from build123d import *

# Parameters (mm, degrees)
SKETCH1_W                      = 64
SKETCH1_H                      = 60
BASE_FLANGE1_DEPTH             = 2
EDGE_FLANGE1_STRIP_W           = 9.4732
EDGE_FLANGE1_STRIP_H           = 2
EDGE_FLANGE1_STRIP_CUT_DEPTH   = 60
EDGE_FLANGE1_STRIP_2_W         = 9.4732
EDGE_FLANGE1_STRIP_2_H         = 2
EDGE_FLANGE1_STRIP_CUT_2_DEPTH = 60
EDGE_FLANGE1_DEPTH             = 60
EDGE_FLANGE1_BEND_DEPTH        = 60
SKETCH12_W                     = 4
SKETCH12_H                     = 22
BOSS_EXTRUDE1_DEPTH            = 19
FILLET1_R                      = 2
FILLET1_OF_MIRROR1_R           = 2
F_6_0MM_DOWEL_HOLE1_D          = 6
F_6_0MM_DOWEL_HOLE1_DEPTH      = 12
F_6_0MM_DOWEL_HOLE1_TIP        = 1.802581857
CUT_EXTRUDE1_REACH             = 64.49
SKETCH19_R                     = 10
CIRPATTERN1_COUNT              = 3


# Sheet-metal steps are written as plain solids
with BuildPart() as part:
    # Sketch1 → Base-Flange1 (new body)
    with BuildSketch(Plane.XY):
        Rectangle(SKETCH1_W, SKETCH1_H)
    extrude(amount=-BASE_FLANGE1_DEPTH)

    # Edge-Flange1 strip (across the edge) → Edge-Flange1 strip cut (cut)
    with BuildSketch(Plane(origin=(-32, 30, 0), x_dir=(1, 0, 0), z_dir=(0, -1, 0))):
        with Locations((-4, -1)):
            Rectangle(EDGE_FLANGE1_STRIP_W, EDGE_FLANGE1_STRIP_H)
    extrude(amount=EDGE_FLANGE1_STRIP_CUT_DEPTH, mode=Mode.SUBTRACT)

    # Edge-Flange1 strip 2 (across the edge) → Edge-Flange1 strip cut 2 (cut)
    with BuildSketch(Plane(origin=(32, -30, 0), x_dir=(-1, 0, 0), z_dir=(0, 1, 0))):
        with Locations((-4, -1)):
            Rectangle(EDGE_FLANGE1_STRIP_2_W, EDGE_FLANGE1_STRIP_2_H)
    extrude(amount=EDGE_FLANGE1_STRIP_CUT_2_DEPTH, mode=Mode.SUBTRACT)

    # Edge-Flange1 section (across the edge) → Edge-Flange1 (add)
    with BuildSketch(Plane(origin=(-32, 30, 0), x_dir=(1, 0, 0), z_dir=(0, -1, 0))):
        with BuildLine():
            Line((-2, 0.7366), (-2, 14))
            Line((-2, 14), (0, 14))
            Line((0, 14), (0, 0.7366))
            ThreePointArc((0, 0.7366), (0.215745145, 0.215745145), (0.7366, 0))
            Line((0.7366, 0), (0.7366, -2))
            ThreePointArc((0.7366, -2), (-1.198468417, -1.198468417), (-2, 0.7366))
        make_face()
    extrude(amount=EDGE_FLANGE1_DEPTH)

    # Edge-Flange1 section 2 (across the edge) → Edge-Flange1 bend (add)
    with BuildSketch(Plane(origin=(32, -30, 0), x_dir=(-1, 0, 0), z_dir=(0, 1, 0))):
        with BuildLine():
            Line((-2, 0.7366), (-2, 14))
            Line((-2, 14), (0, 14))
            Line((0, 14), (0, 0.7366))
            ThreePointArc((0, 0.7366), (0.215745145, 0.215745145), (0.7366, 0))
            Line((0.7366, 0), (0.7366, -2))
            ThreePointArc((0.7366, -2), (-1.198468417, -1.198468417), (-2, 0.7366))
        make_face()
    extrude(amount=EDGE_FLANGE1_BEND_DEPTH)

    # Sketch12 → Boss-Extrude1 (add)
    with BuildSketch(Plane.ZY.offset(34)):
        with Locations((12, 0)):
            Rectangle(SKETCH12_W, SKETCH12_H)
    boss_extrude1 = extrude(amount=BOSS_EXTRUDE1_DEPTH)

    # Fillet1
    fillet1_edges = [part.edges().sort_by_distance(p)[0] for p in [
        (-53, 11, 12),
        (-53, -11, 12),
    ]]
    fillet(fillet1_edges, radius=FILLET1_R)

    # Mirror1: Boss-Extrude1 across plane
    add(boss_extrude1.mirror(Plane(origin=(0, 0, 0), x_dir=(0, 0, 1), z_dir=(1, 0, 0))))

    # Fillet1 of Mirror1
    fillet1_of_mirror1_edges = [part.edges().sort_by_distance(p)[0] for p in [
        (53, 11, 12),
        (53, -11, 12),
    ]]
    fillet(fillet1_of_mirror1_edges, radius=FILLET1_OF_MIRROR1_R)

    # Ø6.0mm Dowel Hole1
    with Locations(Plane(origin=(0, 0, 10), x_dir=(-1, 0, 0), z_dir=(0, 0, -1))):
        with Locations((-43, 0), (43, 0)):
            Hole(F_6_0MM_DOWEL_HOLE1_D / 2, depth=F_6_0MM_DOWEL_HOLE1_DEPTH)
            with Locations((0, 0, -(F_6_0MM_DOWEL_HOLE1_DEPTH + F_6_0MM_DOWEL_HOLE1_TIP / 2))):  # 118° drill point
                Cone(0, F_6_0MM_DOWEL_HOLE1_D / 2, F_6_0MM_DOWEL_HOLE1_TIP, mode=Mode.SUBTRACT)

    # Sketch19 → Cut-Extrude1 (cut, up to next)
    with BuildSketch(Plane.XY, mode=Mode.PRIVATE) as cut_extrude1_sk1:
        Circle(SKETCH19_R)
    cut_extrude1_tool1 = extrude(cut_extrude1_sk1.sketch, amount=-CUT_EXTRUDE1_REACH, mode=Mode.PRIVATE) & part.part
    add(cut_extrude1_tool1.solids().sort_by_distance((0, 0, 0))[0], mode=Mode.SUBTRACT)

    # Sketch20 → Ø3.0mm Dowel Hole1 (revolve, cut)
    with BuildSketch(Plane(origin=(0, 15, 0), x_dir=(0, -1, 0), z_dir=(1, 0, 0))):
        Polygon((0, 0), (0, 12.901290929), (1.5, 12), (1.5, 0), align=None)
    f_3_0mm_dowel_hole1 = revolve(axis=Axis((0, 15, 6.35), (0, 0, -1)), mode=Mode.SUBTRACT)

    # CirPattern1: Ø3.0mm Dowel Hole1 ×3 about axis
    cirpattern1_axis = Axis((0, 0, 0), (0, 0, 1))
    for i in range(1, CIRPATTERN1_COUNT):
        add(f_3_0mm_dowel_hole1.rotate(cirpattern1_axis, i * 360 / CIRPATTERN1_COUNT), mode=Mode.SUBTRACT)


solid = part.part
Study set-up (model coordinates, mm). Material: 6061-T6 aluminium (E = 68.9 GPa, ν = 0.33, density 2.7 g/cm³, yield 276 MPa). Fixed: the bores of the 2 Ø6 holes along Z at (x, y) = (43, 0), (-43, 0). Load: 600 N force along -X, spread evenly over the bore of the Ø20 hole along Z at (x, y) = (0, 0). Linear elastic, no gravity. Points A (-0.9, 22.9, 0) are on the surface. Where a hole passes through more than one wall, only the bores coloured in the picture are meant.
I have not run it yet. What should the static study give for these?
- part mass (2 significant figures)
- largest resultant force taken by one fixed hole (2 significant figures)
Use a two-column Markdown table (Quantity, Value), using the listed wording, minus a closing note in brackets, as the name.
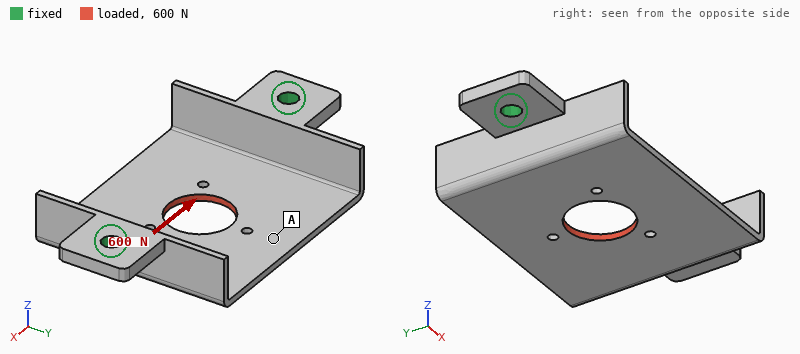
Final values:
| Quantity | Value |
|---|---|
| part mass | 37 g |
| largest resultant force taken by one fixed hole | 300 N |
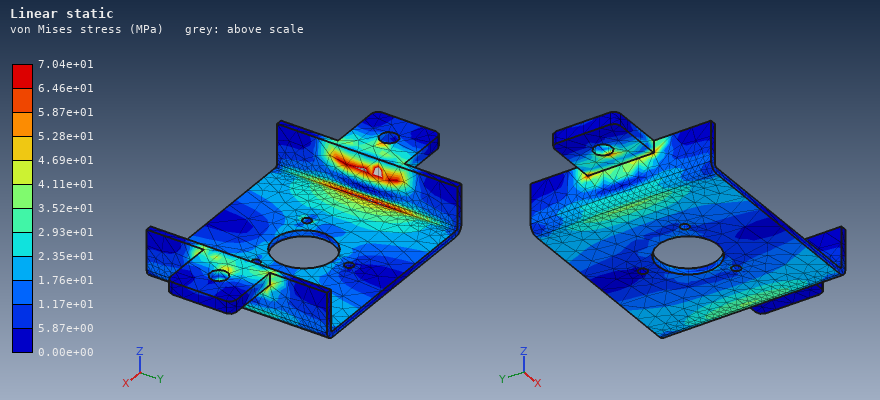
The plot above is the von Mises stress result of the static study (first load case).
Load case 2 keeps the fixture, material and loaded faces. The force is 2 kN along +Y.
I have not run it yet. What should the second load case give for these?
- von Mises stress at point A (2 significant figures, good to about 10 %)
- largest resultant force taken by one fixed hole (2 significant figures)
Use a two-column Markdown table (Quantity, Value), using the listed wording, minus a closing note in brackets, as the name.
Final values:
| Quantity | Value |
|---|---|
| von Mises stress at point A | 18 MPa |
| largest resultant force taken by one fixed hole | 1.0 kN |
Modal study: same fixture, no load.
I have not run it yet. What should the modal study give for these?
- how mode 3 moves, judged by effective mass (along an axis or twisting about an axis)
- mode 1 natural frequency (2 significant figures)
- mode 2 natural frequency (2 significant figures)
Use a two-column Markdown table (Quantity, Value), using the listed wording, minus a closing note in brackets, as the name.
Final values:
| Quantity | Value |
|---|---|
| how mode 3 moves, judged by effective mass | along X |
| mode 1 natural frequency | 2000 Hz |
| mode 2 natural frequency | 2000 Hz |
